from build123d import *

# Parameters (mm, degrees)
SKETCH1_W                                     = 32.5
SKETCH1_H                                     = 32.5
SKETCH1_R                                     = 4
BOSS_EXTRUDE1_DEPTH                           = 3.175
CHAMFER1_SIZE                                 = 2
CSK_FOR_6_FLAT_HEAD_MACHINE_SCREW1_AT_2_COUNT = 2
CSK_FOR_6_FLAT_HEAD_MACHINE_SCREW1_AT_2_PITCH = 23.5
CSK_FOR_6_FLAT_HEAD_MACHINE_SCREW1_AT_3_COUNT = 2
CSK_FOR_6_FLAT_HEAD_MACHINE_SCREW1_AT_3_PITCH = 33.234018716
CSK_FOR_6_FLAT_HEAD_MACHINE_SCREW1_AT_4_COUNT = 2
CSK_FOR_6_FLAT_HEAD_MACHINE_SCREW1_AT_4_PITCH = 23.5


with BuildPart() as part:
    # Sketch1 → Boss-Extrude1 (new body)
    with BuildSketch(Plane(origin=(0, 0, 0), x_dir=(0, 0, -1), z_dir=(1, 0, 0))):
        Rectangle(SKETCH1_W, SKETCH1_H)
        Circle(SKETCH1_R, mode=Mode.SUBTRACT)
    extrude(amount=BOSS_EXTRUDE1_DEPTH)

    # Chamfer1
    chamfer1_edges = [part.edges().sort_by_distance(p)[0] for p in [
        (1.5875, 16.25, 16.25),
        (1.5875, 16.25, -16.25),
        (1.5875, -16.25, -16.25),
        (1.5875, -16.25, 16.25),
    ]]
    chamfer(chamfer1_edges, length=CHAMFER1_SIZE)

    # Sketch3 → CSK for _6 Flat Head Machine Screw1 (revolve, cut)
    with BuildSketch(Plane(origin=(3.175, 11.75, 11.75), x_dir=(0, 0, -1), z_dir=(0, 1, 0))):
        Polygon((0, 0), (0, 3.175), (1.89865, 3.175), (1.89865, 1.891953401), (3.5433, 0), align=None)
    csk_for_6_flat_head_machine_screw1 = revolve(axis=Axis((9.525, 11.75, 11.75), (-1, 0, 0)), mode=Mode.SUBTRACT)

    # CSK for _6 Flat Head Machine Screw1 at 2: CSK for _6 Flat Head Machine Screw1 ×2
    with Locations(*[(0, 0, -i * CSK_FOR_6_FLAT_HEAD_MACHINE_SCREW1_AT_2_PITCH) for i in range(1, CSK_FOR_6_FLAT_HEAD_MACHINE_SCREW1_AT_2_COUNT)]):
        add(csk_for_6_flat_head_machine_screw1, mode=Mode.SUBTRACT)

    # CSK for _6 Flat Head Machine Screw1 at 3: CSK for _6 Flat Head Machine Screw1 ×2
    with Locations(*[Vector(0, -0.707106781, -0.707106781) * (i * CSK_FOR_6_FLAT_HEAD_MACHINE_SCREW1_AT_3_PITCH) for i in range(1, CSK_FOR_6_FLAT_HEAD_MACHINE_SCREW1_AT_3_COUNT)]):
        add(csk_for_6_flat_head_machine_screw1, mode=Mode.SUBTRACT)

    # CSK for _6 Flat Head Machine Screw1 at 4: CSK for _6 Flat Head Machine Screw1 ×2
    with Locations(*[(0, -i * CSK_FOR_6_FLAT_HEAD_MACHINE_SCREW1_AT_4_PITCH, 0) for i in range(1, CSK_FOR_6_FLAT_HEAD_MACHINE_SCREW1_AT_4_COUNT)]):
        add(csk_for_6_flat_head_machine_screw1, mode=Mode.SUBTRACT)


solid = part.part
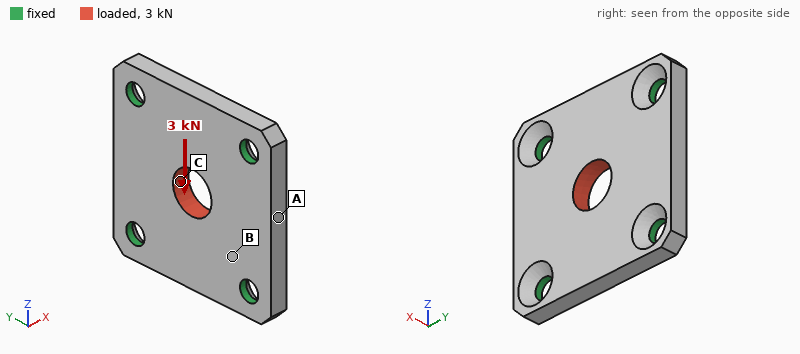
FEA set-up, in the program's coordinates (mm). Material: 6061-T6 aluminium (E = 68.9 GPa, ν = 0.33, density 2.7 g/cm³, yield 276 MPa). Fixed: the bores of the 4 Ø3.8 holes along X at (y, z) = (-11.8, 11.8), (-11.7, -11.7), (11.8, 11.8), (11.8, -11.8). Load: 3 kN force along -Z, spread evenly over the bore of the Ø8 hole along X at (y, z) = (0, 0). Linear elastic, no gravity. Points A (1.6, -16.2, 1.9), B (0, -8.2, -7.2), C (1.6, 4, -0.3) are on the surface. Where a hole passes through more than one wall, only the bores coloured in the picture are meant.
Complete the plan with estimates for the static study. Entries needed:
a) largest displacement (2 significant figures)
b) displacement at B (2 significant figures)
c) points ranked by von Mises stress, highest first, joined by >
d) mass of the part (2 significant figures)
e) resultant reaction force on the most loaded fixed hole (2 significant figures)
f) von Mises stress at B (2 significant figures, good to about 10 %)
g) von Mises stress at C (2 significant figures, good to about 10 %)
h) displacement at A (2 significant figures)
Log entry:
9.3 µm
3.7 µm
C > B > A
7.9 g
810 N
43 MPa
66 MPa
1.6 µm
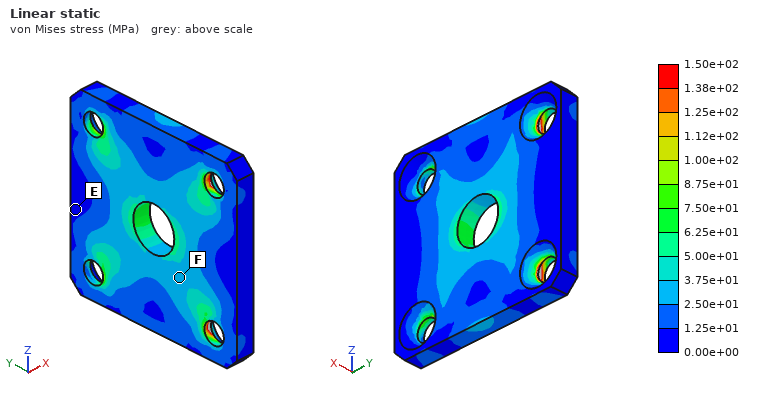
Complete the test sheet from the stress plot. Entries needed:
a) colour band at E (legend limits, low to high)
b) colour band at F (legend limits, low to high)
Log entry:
0.00e+00 to 1.25e+01 MPa
2.50e+01 to 3.75e+01 MPa
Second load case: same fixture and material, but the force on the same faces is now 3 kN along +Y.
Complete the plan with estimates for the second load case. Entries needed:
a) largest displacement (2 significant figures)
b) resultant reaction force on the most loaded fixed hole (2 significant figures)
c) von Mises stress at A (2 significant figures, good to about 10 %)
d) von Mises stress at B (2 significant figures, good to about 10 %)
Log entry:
9.3 µm
810 N
25 MPa
42 MPa
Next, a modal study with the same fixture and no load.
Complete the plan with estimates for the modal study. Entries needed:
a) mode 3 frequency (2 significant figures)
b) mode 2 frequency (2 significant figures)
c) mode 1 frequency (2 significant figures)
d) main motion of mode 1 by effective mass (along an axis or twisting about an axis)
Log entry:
27 kHz
26 kHz
19 kHz
along X
